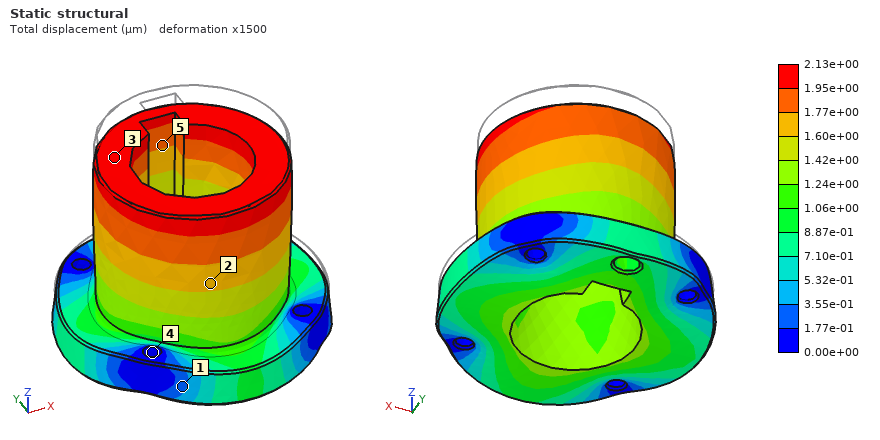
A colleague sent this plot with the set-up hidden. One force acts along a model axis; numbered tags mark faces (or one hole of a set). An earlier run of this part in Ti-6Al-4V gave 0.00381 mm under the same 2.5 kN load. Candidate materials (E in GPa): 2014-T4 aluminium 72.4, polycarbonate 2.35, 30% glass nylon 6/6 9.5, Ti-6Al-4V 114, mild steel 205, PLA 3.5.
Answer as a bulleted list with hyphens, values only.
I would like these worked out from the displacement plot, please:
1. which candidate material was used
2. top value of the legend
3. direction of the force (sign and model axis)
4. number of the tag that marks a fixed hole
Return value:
- mild steel
- 2.13e+00 µm
- -Z
- 4
